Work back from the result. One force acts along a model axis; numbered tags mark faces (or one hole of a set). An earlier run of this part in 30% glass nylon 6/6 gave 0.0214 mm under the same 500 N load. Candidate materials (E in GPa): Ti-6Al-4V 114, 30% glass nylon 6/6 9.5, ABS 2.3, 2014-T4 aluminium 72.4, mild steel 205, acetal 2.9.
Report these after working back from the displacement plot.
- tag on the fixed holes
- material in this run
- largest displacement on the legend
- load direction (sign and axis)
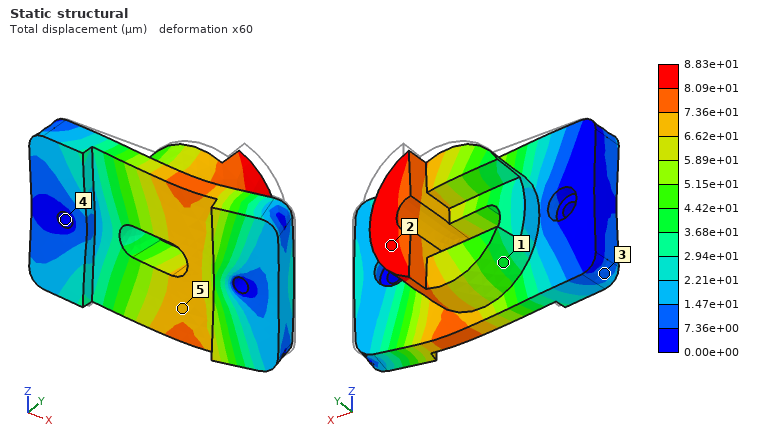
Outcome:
4
ABS
8.83e+01 µm
-Y
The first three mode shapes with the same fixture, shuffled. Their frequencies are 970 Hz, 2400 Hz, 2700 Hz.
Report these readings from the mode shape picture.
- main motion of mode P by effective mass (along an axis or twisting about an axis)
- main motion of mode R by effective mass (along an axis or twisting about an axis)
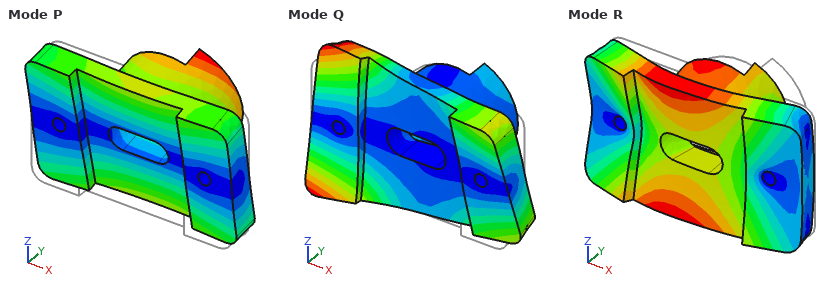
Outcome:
along Z
along Y
